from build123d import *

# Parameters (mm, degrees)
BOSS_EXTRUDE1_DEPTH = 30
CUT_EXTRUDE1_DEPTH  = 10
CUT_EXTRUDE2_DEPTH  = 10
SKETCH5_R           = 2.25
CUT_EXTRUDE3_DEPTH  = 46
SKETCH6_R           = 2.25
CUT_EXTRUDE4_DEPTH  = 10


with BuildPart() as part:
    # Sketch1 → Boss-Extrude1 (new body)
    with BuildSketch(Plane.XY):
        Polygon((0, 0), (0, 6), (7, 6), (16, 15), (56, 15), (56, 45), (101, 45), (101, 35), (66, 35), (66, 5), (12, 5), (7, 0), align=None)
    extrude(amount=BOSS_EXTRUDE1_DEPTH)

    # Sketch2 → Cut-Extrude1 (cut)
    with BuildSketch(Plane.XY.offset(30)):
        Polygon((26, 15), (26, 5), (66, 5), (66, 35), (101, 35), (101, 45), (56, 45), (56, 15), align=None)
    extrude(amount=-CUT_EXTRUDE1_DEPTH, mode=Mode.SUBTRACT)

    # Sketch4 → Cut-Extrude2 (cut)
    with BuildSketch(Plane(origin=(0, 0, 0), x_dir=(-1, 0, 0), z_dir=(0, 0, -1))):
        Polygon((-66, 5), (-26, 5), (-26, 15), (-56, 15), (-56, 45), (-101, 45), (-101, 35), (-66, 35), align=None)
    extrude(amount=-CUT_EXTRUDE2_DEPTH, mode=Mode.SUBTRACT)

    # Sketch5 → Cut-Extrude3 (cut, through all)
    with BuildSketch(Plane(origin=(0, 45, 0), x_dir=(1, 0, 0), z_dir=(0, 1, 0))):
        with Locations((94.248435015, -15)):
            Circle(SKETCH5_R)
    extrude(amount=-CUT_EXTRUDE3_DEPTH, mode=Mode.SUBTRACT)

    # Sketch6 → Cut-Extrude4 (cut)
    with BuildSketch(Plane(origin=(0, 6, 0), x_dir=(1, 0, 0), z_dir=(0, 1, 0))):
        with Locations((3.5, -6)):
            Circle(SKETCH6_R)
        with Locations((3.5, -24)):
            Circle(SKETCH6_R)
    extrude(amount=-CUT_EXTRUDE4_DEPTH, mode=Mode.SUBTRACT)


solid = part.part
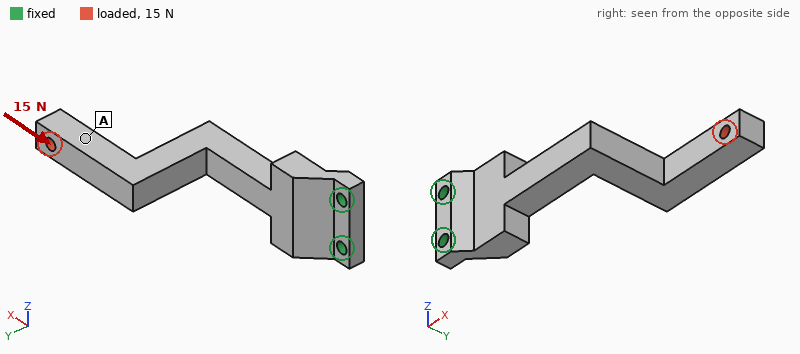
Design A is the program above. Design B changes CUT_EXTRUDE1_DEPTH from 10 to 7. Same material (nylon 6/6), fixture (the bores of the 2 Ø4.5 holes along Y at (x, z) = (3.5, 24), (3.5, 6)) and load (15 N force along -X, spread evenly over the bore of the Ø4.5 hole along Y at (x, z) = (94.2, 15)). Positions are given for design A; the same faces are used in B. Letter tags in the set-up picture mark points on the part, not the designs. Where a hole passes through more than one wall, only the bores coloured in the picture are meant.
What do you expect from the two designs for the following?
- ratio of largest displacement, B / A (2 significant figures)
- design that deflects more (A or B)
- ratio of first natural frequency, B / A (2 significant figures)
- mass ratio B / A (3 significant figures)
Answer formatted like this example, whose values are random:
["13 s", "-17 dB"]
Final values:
["0.90", "A", "0.90", "1.19"]
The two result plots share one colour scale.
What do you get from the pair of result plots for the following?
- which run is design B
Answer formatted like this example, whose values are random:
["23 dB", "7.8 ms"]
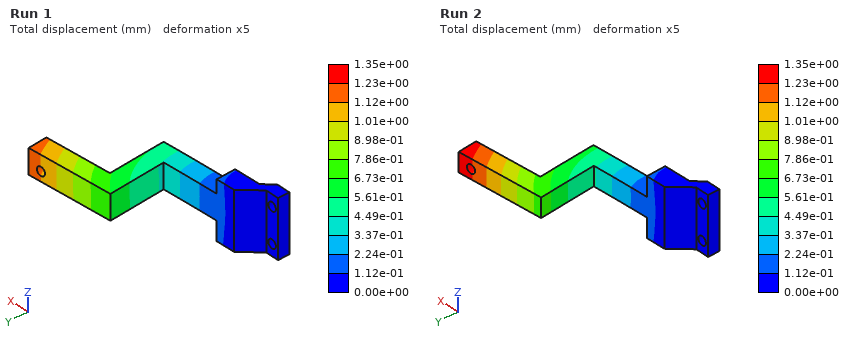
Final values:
["Run 1"]
